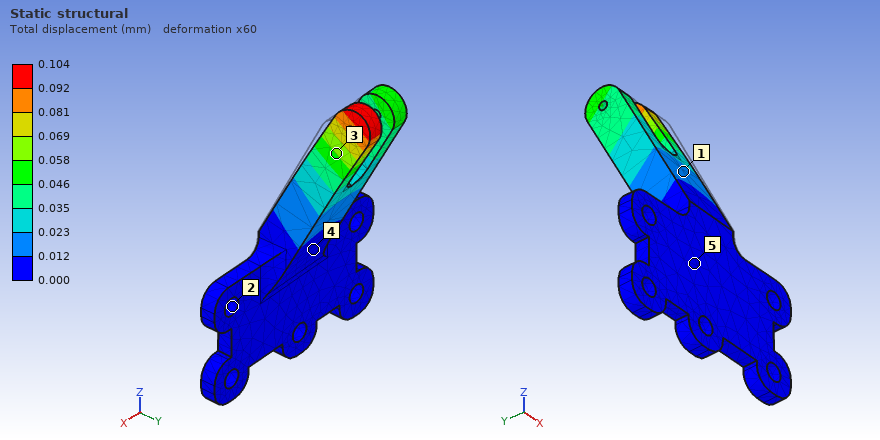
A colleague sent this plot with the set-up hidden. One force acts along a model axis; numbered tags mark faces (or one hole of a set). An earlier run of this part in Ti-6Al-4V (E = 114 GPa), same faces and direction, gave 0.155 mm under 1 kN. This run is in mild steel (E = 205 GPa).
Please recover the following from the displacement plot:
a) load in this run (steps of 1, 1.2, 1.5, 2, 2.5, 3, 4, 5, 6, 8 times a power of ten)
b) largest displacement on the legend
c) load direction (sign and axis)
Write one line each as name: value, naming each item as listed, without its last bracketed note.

load in this run: 1.2 kN
largest displacement on the legend: 0.104 mm
load direction: -X
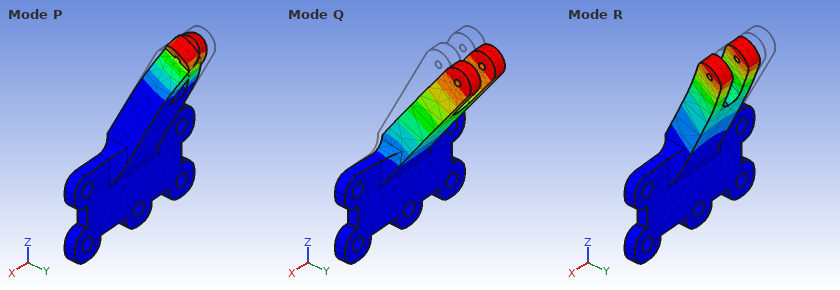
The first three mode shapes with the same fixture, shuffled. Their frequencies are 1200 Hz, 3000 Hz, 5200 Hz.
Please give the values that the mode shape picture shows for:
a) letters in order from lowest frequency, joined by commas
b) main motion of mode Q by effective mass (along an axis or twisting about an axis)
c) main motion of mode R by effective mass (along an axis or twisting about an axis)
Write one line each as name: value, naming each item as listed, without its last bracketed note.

letters in order from lowest frequency, joined by commas: Q, R, P
main motion of mode Q by effective mass: along Y
main motion of mode R by effective mass: along X
